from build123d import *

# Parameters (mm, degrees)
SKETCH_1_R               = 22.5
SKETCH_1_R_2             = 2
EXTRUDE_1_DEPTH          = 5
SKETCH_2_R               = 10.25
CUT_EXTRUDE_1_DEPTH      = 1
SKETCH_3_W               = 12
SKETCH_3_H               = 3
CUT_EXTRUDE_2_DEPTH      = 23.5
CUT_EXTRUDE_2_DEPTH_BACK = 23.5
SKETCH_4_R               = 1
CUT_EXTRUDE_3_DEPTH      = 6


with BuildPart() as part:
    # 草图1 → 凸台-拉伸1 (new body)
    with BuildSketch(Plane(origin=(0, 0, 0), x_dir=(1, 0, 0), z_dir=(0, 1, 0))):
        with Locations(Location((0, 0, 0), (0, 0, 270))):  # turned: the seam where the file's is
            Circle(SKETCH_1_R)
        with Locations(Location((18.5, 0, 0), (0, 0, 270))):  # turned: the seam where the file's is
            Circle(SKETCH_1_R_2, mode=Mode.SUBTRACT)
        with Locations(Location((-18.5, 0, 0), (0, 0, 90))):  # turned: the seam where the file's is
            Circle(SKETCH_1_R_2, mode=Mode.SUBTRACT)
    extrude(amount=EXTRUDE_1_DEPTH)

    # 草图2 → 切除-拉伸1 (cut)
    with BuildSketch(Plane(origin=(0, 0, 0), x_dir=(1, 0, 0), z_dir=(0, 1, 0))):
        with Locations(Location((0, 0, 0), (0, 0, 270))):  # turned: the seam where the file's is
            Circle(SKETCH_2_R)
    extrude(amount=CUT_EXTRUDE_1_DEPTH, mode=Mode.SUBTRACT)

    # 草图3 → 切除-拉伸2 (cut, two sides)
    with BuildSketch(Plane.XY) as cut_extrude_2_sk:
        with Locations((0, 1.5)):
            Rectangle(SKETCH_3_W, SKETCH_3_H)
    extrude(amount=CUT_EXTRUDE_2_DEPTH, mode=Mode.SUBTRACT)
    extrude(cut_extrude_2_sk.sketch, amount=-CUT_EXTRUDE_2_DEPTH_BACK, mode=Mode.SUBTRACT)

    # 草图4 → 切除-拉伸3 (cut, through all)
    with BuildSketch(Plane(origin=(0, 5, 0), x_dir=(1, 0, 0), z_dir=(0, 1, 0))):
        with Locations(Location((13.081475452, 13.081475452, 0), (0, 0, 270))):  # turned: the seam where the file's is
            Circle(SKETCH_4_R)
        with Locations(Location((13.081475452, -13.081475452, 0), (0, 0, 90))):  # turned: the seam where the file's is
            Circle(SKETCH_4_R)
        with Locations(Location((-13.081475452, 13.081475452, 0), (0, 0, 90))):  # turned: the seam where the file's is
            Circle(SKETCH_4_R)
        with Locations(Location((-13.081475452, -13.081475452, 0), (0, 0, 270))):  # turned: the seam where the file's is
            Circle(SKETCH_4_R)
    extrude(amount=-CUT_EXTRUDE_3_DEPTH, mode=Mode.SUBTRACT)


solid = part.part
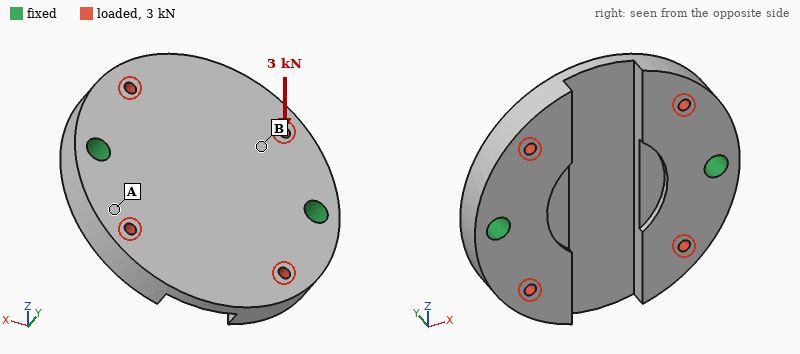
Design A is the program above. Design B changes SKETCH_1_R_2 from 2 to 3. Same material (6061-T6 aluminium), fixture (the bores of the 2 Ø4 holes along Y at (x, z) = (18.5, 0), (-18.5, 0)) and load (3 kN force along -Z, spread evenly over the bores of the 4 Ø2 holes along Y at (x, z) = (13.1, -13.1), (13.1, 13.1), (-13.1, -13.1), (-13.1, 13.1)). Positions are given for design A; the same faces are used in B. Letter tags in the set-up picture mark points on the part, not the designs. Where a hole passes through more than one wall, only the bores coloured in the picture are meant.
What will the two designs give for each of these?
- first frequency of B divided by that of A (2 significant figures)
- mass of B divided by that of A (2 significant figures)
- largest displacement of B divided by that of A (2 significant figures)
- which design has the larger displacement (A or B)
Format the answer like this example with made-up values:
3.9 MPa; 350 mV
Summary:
1.2; 0.97; 0.78; A
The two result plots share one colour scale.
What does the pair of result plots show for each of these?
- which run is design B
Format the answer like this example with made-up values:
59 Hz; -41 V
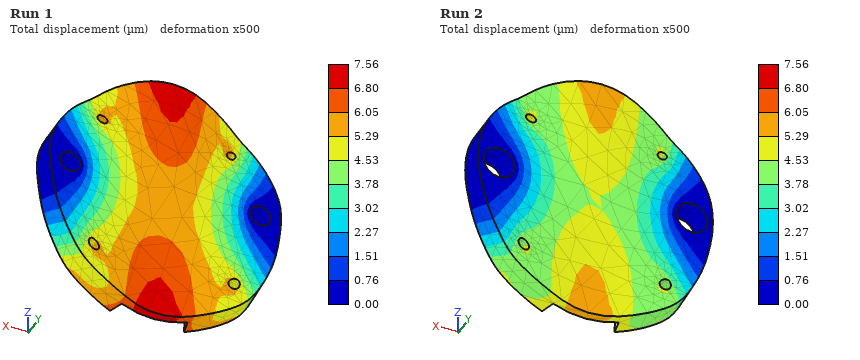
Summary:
Run 2
